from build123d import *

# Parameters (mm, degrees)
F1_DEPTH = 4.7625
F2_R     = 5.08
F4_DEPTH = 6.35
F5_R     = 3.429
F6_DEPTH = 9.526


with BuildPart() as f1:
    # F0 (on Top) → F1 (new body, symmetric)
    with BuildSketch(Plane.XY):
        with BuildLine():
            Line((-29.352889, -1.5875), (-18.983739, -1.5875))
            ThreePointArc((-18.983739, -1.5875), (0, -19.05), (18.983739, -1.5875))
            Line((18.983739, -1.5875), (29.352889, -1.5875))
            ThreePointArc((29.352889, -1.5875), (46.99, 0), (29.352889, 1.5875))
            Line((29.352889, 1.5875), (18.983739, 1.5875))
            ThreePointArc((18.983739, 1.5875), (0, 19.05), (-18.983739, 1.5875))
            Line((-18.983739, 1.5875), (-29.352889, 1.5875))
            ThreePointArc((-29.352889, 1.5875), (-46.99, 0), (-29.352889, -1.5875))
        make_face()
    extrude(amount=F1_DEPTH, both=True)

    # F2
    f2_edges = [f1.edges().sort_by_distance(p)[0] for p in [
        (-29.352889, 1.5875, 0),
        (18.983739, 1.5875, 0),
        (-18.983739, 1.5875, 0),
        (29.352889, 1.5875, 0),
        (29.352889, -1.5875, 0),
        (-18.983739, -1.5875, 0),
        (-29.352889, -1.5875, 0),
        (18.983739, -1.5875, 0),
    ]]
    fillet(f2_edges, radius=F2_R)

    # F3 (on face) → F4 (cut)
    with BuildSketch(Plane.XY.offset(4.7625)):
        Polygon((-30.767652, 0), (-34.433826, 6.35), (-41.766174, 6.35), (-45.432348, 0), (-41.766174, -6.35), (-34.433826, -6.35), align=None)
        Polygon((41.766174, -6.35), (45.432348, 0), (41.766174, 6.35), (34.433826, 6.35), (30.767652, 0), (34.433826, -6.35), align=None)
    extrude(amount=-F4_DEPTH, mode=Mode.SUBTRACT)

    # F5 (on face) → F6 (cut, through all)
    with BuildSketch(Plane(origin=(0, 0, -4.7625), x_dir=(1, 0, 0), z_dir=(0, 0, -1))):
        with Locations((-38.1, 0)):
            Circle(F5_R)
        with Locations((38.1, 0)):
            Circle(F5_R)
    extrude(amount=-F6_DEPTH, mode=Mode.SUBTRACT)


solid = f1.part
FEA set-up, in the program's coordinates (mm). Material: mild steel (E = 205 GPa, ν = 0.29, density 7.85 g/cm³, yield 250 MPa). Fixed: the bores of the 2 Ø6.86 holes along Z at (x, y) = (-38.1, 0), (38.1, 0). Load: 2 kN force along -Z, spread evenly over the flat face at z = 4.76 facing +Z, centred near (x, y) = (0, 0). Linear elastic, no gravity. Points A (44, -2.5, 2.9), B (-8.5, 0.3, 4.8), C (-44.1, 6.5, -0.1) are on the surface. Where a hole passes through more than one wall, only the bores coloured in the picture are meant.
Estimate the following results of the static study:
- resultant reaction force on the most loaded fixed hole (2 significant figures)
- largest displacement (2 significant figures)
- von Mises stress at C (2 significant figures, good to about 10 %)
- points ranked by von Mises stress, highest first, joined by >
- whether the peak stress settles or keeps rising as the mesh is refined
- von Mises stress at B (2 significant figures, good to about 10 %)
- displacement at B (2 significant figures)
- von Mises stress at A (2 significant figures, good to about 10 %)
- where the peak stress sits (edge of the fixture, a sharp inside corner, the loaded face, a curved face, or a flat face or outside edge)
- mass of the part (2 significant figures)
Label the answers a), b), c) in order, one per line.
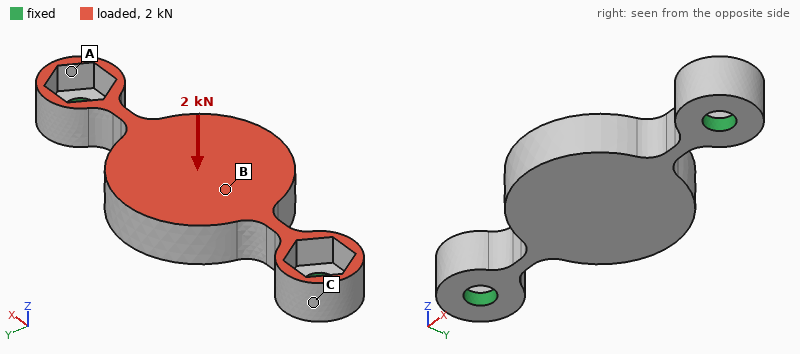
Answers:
a) 1.4 kN
b) 30 µm
c) 23 MPa
d) B > C > A
e) keeps rising
f) 46 MPa
g) 27 µm
h) 14 MPa
i) edge of the fixture
j) 110 g
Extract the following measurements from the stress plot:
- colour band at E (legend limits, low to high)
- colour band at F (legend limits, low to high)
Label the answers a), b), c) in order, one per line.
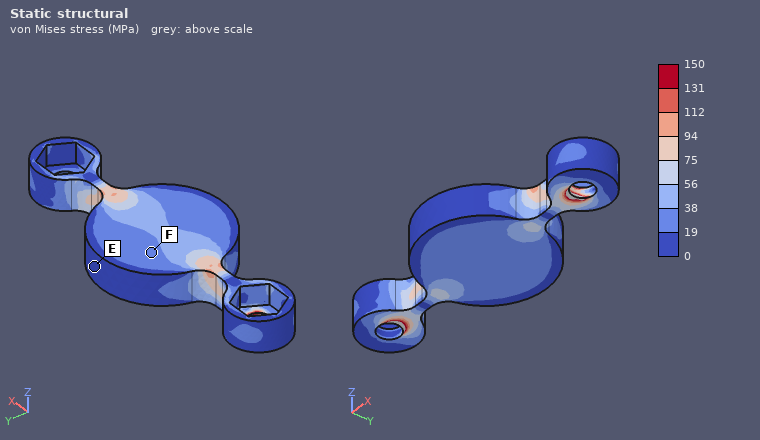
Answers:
a) 0 to 19 MPa
b) 19 to 38 MPa
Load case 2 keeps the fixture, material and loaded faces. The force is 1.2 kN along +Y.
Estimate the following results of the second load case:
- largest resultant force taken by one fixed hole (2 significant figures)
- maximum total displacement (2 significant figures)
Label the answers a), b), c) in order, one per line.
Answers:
a) 600 N
b) 54 µm
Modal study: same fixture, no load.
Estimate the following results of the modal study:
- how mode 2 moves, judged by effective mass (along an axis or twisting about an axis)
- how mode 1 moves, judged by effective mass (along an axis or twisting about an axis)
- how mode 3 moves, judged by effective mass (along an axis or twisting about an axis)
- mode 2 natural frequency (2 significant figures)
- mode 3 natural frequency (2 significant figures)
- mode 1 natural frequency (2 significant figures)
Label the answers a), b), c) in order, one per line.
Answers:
a) along Z
b) twisting about X
c) along Y
d) 4200 Hz
e) 5000 Hz
f) 2500 Hz
